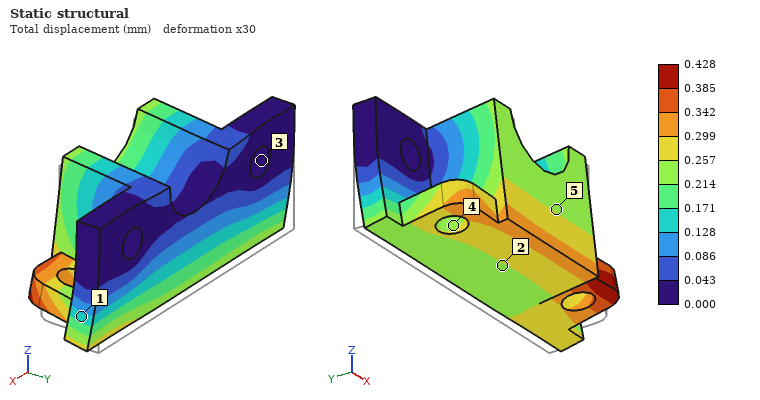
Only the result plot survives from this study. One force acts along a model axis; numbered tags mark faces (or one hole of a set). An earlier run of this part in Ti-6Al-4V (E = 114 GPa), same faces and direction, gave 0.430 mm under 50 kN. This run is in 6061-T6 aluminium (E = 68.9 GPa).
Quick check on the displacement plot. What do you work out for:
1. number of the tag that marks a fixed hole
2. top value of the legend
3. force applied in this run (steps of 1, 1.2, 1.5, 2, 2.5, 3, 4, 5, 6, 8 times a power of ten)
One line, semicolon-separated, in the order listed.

3; 0.428 mm; 30 kN
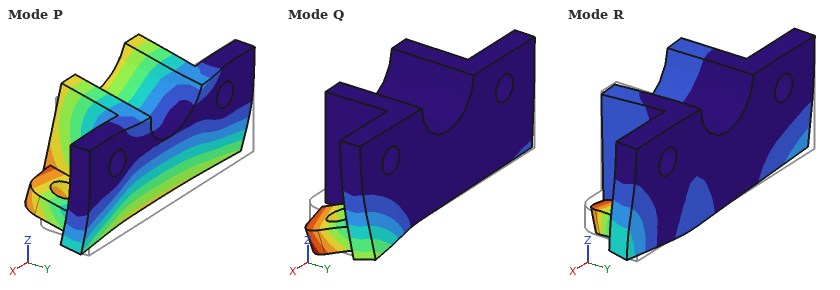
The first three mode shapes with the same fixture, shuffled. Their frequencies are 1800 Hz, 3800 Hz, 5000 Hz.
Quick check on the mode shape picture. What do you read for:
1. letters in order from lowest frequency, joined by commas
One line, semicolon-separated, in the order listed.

P, Q, R
